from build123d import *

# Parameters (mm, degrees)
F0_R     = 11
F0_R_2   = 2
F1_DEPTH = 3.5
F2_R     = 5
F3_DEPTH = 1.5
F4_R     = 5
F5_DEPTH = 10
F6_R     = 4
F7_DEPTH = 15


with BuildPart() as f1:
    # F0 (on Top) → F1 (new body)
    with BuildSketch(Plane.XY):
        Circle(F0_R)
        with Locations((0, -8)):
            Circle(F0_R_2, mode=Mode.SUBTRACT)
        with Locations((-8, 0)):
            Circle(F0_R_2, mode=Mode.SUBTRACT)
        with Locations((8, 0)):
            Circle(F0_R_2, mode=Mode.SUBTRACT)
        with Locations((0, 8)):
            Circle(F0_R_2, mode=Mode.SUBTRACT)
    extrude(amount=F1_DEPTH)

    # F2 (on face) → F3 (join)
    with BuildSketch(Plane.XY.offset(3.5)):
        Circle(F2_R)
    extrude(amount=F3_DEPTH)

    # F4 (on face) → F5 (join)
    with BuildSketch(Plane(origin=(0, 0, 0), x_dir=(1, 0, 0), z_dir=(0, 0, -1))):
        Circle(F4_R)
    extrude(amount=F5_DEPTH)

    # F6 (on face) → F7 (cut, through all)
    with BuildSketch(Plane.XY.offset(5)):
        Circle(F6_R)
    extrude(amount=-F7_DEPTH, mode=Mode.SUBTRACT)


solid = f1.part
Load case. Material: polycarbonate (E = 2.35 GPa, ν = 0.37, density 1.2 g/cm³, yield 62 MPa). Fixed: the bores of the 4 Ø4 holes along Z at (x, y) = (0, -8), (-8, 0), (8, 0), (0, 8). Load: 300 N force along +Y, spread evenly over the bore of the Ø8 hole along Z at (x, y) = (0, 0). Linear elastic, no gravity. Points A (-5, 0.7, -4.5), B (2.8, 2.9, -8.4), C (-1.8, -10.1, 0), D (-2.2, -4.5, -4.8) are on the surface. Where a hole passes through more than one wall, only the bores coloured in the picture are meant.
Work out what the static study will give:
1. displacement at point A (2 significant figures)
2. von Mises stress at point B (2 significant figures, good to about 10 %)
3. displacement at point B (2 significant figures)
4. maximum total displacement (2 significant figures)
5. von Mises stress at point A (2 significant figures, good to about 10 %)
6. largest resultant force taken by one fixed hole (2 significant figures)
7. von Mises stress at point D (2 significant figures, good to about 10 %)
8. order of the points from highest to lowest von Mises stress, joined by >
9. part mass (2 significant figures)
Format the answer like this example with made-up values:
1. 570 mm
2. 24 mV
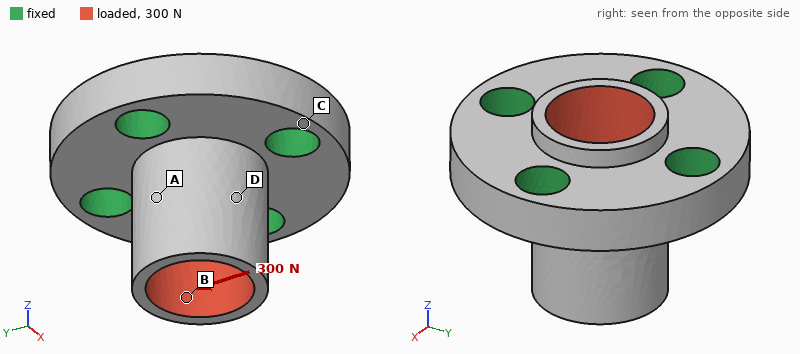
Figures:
1. 0.084 mm
2. 4.4 MPa
3. 0.14 mm
4. 0.17 mm
5. 12 MPa
6. 130 N
7. 7.1 MPa
8. A > D > B > C
9. 1.6 g
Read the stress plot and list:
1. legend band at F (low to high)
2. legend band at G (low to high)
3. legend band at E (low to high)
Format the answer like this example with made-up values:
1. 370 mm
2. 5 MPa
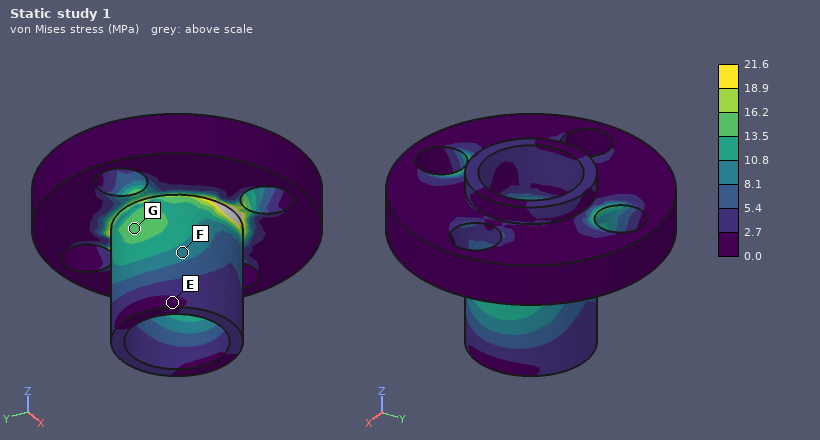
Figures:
1. 8.1 to 10.8 MPa
2. 13.5 to 16.2 MPa
3. 0.0 to 2.7 MPa
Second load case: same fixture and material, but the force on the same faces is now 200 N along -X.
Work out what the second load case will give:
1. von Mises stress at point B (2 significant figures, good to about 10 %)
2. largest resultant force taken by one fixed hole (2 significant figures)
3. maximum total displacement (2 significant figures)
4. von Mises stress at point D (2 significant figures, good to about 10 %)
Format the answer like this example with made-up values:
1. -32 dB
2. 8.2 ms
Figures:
1. 2.9 MPa
2. 85 N
3. 0.11 mm
4. 7.3 MPa
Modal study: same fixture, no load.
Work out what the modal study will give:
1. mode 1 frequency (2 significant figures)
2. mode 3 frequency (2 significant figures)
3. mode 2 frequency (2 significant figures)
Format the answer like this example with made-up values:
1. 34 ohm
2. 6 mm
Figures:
1. 11 kHz
2. 11 kHz
3. 11 kHz
